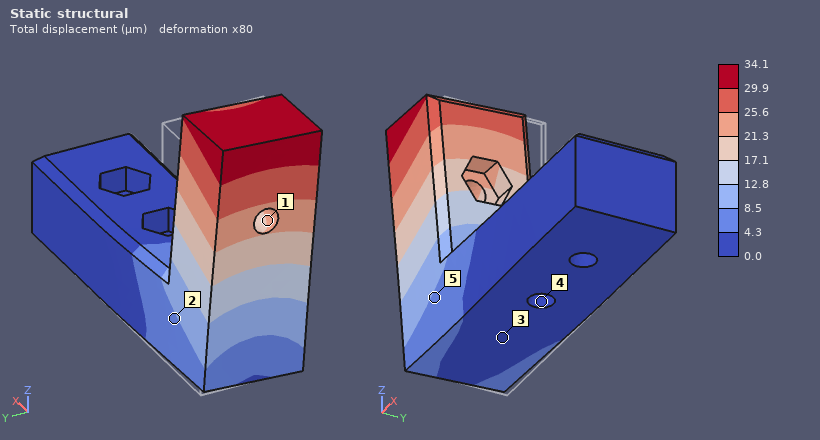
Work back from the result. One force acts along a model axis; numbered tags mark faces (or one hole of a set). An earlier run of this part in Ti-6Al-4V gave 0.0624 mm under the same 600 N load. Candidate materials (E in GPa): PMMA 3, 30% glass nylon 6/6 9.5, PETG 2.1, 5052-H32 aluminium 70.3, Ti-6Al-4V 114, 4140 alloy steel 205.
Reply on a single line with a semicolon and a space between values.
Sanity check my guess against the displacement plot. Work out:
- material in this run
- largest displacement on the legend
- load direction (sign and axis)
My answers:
4140 alloy steel; 34.1 µm; -Y
